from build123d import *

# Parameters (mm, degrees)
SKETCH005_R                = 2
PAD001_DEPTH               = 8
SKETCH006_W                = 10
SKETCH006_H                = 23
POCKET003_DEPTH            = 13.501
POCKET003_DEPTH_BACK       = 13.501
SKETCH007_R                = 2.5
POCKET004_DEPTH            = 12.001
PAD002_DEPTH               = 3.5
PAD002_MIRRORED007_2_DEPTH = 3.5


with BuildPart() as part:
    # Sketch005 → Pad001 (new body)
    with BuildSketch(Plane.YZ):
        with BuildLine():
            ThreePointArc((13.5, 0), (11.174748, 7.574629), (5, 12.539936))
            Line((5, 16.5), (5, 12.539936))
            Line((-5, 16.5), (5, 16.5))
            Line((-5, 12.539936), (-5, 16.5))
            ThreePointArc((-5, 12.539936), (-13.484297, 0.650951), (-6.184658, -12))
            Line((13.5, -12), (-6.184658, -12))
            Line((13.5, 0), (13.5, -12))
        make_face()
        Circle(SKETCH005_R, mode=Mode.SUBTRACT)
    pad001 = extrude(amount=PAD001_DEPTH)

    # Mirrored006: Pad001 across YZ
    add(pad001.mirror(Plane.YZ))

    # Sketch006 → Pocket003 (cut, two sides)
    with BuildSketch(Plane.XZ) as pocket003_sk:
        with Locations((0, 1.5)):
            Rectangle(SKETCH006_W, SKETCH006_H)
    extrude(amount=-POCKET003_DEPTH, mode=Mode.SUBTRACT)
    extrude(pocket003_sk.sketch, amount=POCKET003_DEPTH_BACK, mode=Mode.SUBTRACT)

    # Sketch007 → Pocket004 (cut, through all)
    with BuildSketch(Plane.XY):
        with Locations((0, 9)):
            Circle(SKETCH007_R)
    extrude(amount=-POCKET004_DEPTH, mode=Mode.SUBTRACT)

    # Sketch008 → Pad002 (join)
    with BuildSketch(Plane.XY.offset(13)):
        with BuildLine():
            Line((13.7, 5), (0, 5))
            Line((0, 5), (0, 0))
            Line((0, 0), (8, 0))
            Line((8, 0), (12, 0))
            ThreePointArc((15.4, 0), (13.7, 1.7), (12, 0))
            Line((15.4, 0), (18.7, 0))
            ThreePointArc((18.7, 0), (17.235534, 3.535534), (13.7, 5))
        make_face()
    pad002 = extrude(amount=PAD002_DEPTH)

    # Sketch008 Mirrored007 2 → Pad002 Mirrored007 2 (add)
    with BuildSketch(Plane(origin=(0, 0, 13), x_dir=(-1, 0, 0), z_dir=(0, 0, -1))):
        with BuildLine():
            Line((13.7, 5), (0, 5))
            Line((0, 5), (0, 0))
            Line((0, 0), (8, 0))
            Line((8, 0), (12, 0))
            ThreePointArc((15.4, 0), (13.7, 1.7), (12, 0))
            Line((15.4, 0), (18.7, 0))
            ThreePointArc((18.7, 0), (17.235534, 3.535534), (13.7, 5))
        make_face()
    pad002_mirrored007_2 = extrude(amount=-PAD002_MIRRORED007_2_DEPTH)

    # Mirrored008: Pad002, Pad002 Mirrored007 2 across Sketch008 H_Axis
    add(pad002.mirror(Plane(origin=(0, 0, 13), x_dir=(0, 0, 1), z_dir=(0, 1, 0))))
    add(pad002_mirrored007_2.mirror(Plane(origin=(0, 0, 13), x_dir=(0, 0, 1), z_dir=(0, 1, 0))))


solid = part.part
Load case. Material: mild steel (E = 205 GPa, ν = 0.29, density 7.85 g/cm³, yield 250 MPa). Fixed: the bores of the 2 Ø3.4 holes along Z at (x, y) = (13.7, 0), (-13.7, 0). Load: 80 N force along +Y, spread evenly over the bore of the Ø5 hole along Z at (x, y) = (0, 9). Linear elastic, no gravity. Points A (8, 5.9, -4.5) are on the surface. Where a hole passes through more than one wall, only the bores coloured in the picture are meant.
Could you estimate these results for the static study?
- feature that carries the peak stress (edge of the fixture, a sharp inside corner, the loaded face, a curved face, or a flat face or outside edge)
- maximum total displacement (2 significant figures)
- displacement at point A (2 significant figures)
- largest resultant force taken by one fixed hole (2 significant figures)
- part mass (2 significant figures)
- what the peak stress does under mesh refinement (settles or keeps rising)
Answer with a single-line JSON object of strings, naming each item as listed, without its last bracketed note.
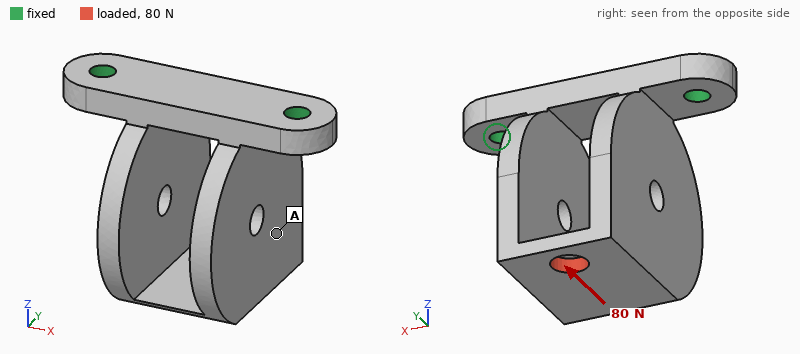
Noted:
{"feature that carries the peak stress": "edge of the fixture", "maximum total displacement": "19 µm", "displacement at point A": "13 µm", "largest resultant force taken by one fixed hole": "40 N", "part mass": "39 g", "what the peak stress does under mesh refinement": "keeps rising"}
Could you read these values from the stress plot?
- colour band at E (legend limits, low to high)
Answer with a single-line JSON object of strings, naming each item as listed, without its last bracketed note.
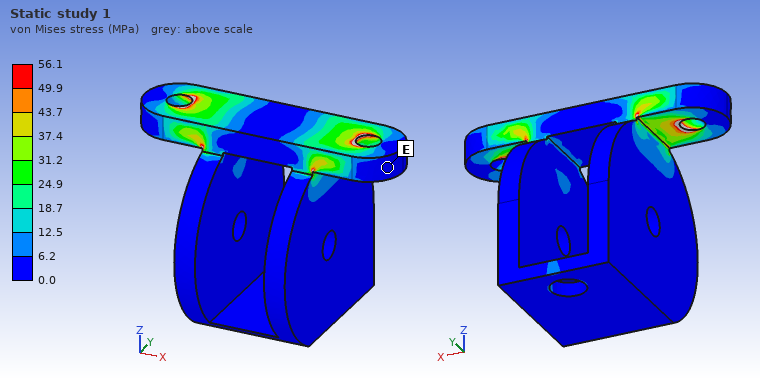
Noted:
{"colour band at E": "0.0 to 6.2 MPa"}
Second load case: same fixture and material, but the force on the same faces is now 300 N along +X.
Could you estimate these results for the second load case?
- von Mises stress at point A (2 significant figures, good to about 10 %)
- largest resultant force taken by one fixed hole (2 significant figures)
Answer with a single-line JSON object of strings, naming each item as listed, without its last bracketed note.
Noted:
{"von Mises stress at point A": "25 MPa", "largest resultant force taken by one fixed hole": "400 N"}
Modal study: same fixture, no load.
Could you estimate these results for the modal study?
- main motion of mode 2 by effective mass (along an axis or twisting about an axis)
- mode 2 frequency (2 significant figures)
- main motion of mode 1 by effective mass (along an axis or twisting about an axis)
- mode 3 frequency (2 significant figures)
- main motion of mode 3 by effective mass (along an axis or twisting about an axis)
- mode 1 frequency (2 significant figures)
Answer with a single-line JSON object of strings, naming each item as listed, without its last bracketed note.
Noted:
{"main motion of mode 2 by effective mass": "along X", "mode 2 frequency": "3500 Hz", "main motion of mode 1 by effective mass": "along Y", "mode 3 frequency": "5700 Hz", "main motion of mode 3 by effective mass": "twisting about Z", "mode 1 frequency": "2800 Hz"}
